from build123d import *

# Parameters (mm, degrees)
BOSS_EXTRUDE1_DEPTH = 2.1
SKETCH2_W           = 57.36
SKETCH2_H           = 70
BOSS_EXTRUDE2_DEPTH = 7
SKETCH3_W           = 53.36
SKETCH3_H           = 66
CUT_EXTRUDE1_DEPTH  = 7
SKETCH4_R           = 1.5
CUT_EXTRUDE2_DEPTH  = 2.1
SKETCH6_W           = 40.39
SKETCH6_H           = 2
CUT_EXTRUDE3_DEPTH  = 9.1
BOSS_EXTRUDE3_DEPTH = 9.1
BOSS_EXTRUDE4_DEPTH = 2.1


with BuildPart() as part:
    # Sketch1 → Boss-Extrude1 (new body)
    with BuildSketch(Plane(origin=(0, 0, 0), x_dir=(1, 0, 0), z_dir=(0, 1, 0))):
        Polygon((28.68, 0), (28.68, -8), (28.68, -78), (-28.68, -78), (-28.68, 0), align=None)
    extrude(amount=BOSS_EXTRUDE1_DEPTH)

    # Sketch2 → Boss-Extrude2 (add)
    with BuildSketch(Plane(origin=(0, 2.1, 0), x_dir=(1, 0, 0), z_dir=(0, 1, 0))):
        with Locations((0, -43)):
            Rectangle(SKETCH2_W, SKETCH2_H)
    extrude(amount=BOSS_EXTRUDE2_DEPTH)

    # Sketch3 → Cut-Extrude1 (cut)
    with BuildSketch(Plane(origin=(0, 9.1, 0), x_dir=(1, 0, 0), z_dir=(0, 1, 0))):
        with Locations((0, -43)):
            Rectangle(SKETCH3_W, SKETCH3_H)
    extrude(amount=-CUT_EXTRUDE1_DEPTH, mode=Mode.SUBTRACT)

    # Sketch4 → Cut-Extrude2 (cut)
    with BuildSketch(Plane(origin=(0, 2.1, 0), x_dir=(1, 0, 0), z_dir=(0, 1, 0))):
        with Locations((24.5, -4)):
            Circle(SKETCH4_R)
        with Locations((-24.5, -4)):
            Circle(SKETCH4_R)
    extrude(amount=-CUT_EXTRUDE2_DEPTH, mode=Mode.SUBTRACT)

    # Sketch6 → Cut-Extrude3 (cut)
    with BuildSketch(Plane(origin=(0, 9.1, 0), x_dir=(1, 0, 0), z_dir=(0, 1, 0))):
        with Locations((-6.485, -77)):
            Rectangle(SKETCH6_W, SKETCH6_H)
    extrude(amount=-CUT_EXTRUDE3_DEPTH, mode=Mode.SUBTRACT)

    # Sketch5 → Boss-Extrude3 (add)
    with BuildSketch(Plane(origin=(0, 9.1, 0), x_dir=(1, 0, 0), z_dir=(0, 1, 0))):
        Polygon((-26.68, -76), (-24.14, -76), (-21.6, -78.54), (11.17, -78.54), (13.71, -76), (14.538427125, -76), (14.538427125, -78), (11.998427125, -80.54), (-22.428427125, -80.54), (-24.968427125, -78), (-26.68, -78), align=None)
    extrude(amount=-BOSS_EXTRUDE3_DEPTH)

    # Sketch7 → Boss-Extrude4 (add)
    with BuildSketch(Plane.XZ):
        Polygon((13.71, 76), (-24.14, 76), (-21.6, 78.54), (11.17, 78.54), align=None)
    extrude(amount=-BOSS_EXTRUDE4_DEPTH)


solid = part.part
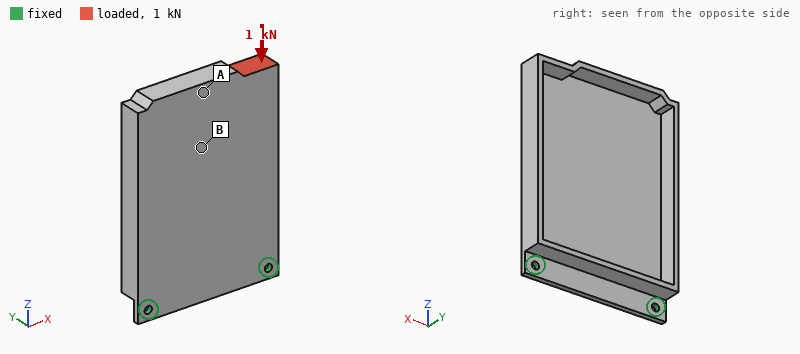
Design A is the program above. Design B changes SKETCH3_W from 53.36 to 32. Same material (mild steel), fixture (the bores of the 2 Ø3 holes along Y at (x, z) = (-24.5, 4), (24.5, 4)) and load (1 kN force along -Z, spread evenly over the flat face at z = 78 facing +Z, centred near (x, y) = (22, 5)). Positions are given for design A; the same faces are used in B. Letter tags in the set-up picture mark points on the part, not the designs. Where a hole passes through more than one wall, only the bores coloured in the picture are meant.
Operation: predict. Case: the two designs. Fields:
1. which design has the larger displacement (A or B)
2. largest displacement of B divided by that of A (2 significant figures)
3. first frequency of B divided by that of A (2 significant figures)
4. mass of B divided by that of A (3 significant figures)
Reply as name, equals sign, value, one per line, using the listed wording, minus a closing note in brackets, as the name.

which design has the larger displacement = A
largest displacement of B divided by that of A = 0.65
first frequency of B divided by that of A = 0.84
mass of B divided by that of A = 1.76
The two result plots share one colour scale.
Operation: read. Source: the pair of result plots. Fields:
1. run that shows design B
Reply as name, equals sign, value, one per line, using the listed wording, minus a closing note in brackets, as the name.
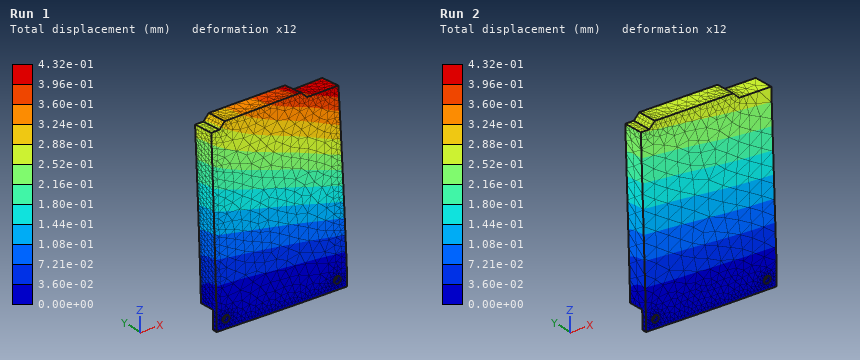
run that shows design B = Run 2
